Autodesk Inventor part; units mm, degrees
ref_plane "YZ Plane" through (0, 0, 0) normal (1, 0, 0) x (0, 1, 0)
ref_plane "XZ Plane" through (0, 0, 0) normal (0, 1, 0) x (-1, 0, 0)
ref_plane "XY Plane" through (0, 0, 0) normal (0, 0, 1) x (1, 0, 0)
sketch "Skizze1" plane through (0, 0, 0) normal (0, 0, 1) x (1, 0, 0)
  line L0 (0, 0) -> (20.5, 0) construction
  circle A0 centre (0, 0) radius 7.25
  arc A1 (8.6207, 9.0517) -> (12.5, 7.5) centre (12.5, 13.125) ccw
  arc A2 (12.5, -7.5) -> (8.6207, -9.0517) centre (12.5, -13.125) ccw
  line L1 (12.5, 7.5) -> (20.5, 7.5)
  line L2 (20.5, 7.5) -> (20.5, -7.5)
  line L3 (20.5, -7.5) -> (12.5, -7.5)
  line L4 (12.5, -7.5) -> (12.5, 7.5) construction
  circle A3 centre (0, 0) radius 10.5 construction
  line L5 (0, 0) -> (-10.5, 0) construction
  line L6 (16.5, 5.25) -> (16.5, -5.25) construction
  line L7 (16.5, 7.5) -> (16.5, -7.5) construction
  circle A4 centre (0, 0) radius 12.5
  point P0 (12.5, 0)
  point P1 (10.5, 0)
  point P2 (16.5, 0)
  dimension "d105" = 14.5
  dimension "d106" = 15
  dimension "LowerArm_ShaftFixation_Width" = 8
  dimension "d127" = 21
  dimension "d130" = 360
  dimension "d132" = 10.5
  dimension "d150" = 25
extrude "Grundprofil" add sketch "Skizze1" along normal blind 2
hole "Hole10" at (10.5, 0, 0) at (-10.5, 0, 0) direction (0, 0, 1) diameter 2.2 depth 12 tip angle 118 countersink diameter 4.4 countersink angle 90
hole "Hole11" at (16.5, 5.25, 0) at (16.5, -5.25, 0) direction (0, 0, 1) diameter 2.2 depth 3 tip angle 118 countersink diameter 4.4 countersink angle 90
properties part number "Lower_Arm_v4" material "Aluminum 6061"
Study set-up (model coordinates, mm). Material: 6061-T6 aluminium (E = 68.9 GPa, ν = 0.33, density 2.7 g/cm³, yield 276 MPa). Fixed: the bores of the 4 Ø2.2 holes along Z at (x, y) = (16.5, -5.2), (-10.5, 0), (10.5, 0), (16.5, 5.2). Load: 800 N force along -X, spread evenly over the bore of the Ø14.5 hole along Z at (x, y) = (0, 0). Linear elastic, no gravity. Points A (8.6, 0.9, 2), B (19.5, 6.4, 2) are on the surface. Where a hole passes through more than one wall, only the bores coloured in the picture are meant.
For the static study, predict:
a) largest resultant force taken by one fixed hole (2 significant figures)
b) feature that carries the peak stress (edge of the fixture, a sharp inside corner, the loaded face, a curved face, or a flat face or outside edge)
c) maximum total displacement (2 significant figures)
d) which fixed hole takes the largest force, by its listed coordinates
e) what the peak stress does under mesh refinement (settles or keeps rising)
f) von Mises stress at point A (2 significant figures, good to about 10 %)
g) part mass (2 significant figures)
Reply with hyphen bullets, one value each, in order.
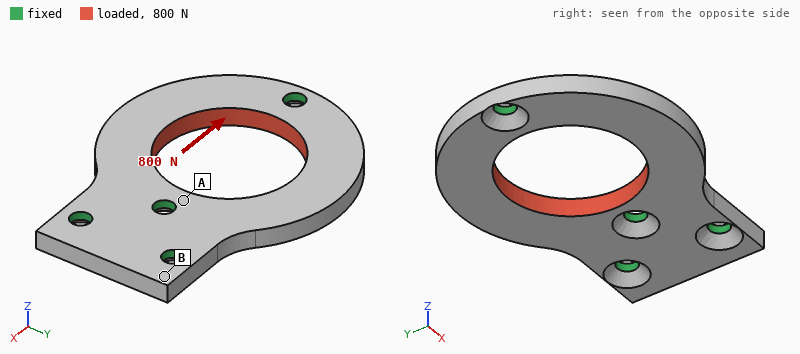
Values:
- 310 N
- edge of the fixture
- 6.1 µm
- (-10.5, 0)
- keeps rising
- 22 MPa
- 2.3 g
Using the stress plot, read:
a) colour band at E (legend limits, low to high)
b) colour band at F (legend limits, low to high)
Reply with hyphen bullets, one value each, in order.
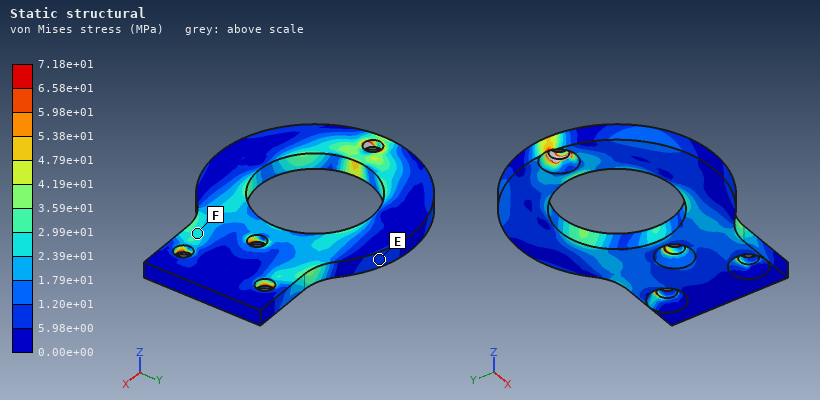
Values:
- 5.98e+00 to 1.20e+01 MPa
- 2.39e+01 to 2.99e+01 MPa
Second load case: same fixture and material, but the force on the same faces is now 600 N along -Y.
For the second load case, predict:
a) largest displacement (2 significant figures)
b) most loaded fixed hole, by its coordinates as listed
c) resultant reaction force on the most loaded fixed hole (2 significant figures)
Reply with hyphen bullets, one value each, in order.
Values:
- 12 µm
- (-10.5, 0)
- 300 N
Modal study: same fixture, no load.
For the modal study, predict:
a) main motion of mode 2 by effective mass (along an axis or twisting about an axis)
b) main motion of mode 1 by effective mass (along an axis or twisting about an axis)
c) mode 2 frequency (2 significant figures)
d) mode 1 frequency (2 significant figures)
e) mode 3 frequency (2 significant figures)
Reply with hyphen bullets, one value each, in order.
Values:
- along Z
- twisting about X
- 8800 Hz
- 7700 Hz
- 22 kHz
